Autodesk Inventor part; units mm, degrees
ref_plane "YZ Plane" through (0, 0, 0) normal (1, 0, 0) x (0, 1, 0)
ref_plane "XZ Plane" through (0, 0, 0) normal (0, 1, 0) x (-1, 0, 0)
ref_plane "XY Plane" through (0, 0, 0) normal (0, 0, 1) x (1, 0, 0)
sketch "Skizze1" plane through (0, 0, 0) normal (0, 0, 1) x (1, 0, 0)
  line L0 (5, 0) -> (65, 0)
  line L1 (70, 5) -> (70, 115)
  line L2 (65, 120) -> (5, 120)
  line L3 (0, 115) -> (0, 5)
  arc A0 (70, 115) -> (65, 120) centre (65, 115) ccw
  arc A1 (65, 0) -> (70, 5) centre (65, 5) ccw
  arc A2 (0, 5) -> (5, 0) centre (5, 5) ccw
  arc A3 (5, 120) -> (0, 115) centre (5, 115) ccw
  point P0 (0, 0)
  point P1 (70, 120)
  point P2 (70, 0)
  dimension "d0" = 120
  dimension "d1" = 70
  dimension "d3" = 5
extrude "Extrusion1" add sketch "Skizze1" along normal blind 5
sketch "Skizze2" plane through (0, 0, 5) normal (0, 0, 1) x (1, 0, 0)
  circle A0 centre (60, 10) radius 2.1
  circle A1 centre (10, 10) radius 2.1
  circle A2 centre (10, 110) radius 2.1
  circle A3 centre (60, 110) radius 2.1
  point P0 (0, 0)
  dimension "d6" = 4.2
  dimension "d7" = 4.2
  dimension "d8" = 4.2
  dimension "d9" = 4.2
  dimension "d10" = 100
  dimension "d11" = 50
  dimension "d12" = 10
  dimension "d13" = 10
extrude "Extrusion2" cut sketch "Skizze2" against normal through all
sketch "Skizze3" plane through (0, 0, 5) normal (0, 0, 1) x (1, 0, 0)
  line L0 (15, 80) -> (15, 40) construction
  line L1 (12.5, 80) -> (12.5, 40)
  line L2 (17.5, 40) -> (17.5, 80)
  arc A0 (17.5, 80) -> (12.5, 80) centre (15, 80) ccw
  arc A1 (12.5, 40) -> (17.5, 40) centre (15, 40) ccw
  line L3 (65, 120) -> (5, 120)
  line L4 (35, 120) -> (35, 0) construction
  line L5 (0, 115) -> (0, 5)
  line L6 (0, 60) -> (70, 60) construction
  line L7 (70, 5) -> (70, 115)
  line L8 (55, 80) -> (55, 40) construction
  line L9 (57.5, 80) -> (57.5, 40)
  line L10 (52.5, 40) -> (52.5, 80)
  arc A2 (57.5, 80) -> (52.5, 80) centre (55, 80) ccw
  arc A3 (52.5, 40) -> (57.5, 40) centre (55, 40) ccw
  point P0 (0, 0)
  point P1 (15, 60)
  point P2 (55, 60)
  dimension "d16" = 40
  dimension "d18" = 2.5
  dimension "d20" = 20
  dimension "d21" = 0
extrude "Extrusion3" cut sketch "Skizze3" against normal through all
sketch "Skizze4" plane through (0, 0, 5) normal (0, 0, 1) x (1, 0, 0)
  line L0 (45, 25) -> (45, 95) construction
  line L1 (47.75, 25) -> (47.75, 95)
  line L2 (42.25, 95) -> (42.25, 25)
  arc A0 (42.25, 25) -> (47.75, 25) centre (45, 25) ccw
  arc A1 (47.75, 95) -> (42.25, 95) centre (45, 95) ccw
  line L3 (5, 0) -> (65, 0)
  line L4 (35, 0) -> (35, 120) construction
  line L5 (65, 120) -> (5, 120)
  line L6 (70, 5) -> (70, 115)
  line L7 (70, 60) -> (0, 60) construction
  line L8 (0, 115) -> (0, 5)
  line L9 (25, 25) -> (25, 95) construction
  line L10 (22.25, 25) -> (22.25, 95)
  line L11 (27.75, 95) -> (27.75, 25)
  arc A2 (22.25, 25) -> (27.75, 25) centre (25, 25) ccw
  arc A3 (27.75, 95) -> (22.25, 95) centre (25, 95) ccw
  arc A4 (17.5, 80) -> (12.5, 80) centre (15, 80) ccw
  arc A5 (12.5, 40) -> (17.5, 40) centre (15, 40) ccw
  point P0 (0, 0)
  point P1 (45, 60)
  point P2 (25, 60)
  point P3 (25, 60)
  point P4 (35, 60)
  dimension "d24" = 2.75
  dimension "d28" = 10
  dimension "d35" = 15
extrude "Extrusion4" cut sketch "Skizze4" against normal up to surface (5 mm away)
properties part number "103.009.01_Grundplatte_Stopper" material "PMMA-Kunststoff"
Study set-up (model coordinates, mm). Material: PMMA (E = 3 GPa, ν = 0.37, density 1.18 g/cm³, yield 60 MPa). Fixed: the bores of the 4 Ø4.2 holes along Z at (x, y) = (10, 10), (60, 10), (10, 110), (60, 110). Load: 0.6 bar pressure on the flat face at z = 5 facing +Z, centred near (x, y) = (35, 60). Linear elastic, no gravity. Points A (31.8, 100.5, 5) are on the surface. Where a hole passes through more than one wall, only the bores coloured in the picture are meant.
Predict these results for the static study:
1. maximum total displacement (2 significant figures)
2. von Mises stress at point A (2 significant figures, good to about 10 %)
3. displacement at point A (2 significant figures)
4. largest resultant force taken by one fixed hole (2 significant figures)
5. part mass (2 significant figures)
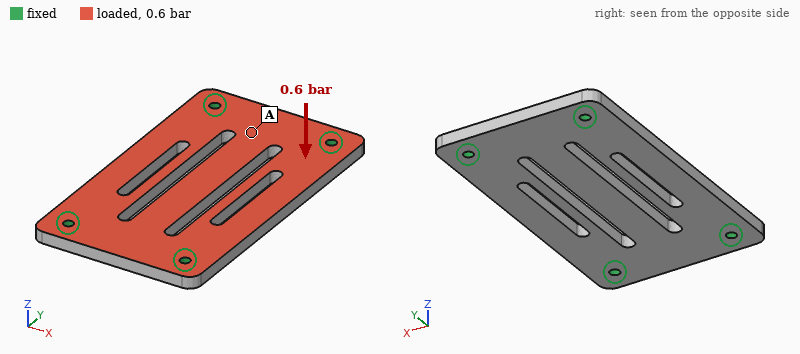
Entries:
0.69 mm
4.8 MPa
0.18 mm
110 N
42 g
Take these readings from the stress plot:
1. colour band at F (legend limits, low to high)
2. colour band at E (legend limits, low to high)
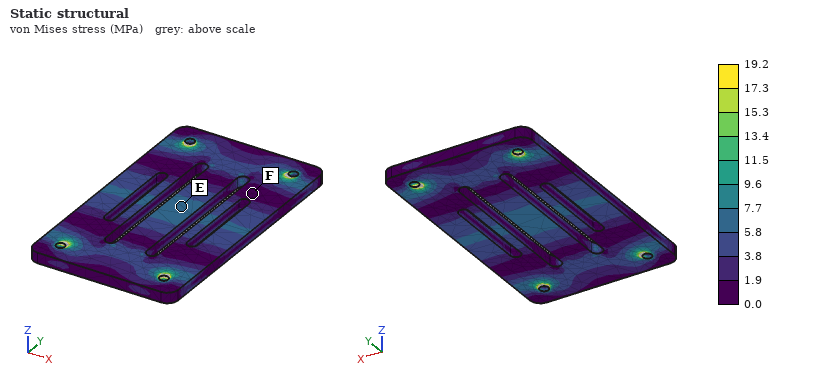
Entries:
0.0 to 1.9 MPa
5.8 to 7.7 MPa
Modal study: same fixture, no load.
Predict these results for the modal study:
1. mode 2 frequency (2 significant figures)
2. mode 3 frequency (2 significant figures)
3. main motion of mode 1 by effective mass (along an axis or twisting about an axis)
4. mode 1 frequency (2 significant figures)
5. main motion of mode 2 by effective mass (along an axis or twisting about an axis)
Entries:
910 Hz
970 Hz
along Z
760 Hz
twisting about Y
